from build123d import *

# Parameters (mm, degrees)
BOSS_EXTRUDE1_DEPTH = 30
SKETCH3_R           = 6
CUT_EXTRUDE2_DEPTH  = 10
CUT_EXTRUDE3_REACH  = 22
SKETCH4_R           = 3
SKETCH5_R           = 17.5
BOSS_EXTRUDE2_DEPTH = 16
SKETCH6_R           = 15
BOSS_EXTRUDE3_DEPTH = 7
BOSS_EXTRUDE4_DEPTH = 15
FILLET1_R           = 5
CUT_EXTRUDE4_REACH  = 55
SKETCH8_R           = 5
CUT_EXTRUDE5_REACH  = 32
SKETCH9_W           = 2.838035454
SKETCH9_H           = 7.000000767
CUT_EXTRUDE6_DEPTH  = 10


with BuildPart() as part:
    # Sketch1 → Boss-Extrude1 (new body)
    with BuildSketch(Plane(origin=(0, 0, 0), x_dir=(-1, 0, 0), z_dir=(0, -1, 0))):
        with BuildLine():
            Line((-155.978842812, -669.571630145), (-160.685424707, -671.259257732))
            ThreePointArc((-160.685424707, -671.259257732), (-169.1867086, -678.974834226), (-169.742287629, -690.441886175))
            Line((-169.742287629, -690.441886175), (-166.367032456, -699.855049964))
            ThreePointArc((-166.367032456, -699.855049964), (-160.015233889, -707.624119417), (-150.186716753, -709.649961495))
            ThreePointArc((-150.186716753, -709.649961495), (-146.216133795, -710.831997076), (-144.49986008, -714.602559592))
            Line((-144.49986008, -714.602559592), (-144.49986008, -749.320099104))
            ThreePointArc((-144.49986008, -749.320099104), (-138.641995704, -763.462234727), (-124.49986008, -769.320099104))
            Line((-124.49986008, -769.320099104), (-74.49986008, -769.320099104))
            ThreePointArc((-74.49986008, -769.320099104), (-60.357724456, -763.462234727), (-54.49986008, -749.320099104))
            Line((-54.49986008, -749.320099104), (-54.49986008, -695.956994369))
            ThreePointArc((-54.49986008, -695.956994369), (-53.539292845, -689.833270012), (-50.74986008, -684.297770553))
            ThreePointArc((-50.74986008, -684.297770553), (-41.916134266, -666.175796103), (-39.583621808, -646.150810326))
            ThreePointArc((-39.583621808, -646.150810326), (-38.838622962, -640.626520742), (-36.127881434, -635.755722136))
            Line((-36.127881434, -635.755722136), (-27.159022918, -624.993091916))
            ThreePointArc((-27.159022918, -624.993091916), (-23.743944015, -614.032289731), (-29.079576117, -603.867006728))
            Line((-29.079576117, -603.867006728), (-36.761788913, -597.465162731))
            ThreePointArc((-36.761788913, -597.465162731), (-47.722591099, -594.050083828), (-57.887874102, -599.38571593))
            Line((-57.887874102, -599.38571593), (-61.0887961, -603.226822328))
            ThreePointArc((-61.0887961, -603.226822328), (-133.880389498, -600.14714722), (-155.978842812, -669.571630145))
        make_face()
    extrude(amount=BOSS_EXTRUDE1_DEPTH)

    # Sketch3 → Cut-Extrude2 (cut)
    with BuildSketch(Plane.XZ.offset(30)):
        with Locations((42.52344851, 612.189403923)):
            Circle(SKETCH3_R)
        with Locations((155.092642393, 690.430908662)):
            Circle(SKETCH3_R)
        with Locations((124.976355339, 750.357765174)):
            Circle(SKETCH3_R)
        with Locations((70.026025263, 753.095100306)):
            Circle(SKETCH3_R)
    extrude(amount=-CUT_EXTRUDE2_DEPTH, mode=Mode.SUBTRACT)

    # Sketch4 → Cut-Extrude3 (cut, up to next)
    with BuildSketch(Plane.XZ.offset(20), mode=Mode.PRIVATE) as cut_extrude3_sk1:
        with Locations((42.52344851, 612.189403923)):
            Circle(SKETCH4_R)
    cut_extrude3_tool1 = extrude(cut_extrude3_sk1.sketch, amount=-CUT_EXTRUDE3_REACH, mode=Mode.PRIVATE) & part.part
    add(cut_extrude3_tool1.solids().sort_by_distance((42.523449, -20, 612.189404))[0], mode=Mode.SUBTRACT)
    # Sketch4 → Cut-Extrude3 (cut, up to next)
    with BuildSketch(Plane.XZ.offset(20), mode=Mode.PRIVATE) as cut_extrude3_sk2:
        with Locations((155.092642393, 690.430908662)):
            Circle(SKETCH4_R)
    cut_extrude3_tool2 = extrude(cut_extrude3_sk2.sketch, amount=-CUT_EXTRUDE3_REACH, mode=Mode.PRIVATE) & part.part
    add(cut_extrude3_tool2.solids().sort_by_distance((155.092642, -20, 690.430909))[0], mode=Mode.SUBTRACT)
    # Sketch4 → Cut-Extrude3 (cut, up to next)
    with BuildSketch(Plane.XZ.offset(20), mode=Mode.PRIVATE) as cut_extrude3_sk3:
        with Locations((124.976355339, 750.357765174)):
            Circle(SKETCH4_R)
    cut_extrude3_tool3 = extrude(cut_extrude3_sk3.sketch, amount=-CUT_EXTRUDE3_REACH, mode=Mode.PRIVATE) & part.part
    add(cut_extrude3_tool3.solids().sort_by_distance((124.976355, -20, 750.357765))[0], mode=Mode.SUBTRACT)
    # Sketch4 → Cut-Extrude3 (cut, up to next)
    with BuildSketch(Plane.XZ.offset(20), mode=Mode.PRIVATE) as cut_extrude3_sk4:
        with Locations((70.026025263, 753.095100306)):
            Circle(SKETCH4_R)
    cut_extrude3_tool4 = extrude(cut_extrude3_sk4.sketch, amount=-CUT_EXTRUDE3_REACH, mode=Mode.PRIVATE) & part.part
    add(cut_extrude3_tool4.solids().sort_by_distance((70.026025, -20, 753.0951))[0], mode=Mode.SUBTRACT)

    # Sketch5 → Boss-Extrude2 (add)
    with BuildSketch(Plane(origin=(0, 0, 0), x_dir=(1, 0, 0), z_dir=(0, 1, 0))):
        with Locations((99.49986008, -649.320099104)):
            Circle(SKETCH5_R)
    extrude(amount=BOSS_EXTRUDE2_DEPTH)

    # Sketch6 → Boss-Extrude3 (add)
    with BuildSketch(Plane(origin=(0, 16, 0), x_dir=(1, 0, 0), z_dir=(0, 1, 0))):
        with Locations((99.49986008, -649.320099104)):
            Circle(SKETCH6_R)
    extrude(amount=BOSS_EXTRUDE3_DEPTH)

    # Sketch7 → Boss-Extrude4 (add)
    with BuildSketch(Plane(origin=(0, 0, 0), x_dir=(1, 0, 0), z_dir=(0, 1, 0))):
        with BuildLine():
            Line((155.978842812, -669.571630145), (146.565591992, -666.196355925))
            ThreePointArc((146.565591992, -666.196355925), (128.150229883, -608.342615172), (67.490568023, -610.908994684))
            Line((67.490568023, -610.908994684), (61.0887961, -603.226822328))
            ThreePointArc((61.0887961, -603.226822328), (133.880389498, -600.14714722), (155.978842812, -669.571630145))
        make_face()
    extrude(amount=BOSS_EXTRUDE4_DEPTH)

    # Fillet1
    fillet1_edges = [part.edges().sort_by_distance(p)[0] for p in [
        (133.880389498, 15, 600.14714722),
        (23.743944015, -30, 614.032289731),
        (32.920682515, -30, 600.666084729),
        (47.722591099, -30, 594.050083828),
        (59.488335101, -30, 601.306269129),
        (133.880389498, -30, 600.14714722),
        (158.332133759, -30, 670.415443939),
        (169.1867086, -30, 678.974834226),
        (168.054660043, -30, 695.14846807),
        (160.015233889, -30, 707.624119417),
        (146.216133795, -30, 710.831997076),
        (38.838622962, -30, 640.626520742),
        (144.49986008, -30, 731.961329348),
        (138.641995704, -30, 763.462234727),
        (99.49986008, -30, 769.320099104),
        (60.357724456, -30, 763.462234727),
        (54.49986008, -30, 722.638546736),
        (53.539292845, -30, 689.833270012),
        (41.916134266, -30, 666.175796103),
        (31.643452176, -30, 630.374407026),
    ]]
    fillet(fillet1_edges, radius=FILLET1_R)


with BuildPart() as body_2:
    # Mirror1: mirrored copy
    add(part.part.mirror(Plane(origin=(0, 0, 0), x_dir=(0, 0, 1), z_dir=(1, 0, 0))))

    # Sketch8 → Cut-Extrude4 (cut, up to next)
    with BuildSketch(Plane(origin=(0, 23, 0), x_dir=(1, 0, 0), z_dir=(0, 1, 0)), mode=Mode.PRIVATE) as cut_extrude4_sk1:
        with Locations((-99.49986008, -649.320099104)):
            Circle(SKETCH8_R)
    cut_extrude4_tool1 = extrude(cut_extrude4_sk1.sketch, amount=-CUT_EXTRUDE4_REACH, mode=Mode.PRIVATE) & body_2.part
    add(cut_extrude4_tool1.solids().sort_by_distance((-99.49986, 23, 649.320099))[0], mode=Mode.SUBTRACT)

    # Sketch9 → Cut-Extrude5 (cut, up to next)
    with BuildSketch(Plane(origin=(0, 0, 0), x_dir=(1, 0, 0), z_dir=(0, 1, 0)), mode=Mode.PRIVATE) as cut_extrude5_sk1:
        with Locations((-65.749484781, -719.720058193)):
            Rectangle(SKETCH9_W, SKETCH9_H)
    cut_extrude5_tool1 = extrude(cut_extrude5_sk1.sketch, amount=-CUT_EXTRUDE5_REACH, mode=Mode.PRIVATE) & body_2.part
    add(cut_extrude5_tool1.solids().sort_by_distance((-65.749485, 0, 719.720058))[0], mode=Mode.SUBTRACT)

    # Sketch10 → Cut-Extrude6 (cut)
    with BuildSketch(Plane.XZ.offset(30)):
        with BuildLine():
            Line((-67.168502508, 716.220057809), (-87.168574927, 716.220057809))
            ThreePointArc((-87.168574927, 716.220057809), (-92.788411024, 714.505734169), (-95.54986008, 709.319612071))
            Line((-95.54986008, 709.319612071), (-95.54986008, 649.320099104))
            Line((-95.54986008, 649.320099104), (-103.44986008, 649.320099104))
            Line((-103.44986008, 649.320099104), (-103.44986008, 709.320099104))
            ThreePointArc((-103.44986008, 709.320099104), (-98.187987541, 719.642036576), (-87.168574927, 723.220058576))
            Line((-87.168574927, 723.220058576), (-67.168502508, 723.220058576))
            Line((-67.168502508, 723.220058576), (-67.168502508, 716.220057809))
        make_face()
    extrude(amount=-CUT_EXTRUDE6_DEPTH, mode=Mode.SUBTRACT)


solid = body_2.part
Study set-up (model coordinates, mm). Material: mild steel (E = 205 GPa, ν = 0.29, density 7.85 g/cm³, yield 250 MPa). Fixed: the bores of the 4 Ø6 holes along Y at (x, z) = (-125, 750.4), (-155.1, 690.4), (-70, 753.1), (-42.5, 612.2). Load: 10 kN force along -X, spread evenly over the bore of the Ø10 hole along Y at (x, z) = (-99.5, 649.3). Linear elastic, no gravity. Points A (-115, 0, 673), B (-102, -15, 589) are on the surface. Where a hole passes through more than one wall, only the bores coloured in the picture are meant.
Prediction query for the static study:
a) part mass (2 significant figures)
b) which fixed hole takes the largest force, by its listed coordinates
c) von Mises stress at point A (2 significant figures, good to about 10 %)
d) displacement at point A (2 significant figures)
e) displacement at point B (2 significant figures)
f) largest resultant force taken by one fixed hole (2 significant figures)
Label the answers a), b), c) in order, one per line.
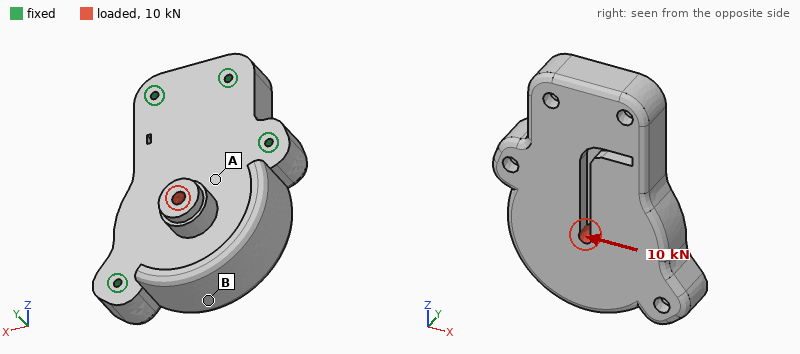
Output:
a) 4.6 kg
b) (-42.5, 612.2)
c) 7.9 MPa
d) 1.9 µm
e) 2.3 µm
f) 5.0 kN
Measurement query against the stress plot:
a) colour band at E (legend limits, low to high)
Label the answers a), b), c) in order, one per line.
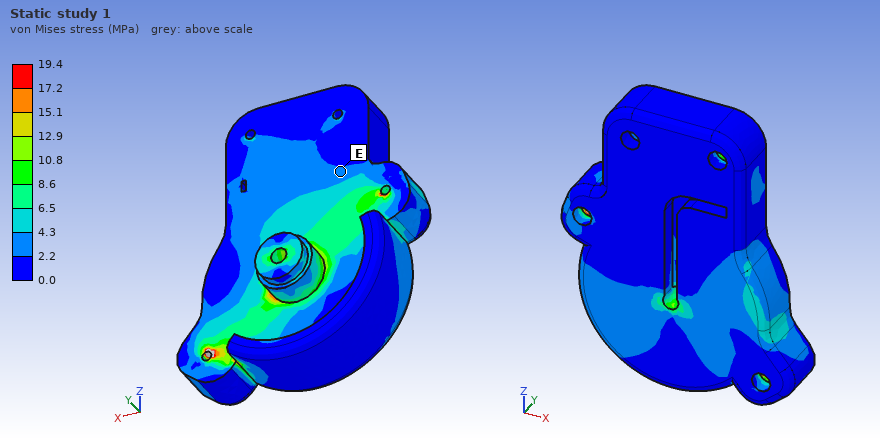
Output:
a) 2.2 to 4.3 MPa
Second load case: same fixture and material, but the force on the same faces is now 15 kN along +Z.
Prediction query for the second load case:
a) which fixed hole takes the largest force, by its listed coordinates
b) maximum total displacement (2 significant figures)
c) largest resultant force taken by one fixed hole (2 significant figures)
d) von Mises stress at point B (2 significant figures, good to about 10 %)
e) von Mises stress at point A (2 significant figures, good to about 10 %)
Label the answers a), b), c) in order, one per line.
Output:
a) (-155.1, 690.4)
b) 10 µm
c) 4.4 kN
d) 3.4 MPa
e) 13 MPa
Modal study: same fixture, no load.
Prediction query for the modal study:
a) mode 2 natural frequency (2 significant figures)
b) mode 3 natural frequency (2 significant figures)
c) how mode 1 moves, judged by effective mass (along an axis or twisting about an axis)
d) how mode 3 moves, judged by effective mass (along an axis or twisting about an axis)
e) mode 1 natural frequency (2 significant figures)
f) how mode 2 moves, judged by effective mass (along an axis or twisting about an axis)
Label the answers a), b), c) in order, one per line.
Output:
a) 4800 Hz
b) 7200 Hz
c) along Y
d) along X
e) 2900 Hz
f) along Y
